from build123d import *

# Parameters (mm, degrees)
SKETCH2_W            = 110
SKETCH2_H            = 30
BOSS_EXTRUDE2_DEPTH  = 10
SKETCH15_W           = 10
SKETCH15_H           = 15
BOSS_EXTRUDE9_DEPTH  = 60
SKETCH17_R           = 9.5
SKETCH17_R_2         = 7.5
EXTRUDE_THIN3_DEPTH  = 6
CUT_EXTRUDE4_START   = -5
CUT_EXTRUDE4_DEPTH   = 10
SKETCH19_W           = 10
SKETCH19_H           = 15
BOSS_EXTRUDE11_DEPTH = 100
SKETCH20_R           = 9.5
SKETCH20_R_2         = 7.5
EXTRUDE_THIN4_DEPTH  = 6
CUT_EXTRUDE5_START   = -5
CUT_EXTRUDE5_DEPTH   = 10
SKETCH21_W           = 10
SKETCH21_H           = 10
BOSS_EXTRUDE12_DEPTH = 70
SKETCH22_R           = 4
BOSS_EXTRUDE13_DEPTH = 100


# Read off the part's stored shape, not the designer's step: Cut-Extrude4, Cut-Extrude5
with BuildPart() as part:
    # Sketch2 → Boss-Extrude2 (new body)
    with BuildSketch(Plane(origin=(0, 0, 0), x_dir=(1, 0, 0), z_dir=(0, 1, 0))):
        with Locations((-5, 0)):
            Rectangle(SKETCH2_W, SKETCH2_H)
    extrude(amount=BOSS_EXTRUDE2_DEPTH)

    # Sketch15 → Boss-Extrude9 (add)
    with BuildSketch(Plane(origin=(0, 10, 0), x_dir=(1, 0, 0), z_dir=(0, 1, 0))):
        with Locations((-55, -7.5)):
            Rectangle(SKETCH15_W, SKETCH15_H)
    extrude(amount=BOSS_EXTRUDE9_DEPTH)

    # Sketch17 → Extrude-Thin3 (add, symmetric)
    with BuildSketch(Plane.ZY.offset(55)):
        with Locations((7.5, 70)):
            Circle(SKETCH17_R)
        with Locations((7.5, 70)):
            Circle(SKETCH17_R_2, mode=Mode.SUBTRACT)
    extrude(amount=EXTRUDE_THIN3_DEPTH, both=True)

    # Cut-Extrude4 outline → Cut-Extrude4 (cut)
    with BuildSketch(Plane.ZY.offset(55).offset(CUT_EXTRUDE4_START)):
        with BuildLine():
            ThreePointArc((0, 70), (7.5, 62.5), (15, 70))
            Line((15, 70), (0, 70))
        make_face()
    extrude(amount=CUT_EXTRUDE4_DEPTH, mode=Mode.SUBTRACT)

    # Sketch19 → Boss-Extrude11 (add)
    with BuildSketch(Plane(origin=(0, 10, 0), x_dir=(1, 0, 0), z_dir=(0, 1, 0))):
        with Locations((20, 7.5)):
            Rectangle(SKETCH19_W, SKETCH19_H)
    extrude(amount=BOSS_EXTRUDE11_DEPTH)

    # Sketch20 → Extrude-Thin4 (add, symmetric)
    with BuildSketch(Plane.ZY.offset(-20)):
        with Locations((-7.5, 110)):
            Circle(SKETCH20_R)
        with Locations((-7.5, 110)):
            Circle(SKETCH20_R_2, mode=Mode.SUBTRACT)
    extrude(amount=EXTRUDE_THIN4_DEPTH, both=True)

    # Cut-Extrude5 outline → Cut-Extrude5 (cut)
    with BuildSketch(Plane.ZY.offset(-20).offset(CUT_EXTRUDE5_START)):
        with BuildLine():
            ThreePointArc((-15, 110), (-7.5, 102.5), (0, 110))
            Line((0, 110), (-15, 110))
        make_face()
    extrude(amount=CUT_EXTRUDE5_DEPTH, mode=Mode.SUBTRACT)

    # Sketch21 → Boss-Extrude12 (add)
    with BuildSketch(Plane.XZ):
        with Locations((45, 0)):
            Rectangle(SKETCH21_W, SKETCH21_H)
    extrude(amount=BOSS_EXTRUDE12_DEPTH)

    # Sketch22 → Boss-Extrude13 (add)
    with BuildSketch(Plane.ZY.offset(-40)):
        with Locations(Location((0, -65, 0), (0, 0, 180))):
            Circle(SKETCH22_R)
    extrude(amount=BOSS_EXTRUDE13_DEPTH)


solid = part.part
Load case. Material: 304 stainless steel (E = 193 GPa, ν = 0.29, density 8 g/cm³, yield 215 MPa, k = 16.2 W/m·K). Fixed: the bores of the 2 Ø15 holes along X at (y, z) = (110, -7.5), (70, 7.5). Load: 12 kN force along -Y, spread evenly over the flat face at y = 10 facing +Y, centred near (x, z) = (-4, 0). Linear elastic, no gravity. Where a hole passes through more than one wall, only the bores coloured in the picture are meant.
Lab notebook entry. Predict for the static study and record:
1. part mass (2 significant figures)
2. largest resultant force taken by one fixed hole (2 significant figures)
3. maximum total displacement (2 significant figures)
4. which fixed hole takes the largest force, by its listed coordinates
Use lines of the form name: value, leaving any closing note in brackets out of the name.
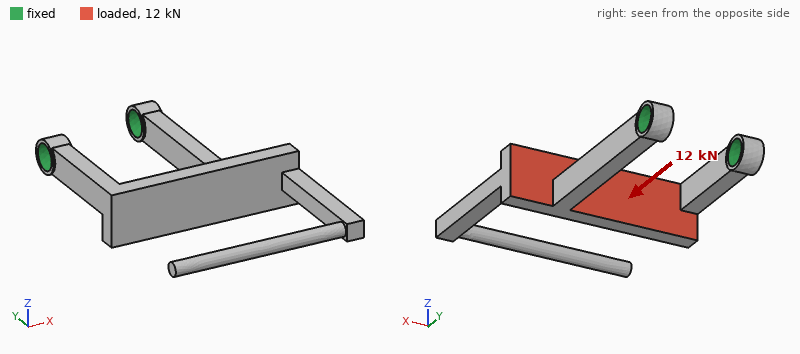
part mass: 550 g
largest resultant force taken by one fixed hole: 8.1 kN
maximum total displacement: 0.55 mm
which fixed hole takes the largest force, by its listed coordinates: (110, -7.5)
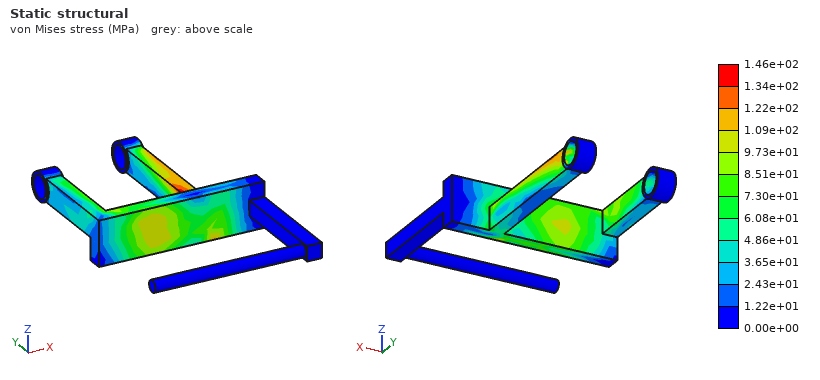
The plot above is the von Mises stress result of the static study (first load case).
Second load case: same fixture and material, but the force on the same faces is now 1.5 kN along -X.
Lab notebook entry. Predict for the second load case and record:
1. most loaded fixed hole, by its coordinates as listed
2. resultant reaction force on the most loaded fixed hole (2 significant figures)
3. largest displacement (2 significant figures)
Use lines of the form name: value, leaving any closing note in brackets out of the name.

most loaded fixed hole, by its coordinates as listed: (70, 7.5)
resultant reaction force on the most loaded fixed hole: 1.3 kN
largest displacement: 0.16 mm
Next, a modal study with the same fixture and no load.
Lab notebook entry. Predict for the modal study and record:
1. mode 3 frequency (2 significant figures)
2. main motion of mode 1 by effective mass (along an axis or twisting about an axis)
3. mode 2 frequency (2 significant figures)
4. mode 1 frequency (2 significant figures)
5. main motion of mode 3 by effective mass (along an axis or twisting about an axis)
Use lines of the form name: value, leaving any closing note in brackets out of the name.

mode 3 frequency: 480 Hz
main motion of mode 1 by effective mass: along Z
mode 2 frequency: 370 Hz
mode 1 frequency: 300 Hz
main motion of mode 3 by effective mass: along Z
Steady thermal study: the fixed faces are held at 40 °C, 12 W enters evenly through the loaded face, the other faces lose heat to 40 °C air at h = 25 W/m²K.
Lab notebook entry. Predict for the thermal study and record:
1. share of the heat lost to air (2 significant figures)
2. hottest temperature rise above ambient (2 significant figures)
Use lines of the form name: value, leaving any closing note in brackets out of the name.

share of the heat lost to air: 86 %
hottest temperature rise above ambient: 48 K
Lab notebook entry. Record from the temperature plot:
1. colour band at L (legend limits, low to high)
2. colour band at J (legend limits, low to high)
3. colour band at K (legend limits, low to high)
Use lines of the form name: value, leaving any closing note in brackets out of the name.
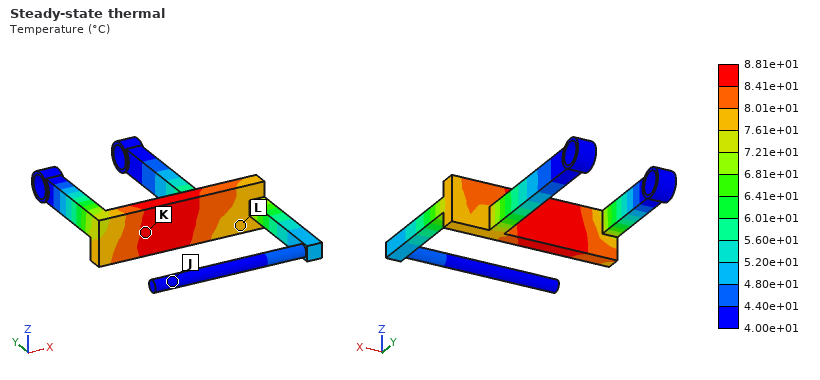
colour band at L: 7.61e+01 to 8.01e+01 °C
colour band at J: 4.00e+01 to 4.40e+01 °C
colour band at K: 8.41e+01 to 8.81e+01 °C
